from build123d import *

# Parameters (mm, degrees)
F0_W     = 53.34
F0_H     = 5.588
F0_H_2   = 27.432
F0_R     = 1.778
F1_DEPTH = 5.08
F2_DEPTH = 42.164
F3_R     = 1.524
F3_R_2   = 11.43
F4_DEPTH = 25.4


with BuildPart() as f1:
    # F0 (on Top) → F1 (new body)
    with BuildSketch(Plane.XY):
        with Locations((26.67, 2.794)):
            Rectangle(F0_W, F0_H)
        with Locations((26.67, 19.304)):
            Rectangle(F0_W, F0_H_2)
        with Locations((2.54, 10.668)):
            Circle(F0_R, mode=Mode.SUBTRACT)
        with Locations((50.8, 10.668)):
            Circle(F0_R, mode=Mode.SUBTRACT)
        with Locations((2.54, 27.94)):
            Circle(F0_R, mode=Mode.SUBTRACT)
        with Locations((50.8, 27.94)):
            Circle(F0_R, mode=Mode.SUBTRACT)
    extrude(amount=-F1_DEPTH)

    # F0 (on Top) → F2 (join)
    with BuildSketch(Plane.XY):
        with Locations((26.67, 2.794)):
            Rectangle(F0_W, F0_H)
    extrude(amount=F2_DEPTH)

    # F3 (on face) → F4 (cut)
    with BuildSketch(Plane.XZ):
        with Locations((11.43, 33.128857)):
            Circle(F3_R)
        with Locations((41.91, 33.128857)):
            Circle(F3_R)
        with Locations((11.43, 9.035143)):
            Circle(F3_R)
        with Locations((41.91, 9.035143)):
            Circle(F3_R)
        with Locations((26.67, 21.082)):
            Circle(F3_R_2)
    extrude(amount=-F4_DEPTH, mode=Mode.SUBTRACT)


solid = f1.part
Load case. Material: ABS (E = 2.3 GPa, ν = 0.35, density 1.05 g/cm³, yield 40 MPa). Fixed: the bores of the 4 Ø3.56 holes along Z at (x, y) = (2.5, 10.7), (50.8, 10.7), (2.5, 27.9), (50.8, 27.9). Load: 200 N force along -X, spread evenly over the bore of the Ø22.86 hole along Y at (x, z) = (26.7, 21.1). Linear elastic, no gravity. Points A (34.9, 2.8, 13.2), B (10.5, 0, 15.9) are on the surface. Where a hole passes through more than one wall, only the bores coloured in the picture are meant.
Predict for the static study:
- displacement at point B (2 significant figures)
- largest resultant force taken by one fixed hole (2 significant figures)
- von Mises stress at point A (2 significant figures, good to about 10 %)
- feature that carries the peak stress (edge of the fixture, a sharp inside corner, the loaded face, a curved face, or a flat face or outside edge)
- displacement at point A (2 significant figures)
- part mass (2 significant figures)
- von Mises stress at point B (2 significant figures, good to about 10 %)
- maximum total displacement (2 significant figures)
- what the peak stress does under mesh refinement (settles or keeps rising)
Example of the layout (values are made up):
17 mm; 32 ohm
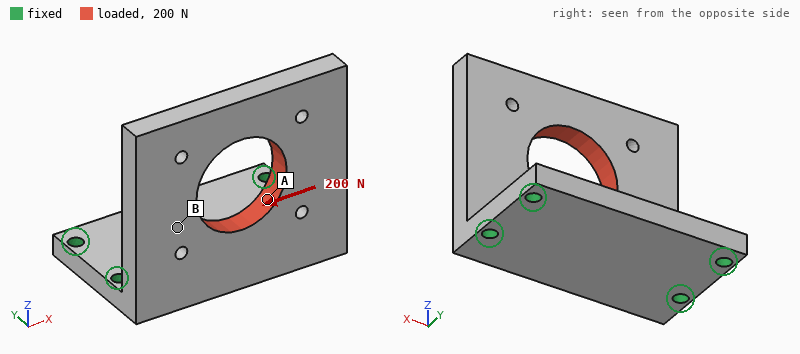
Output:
0.081 mm; 140 N; 3.8 MPa; edge of the fixture; 0.060 mm; 20 g; 1.2 MPa; 0.20 mm; keeps rising
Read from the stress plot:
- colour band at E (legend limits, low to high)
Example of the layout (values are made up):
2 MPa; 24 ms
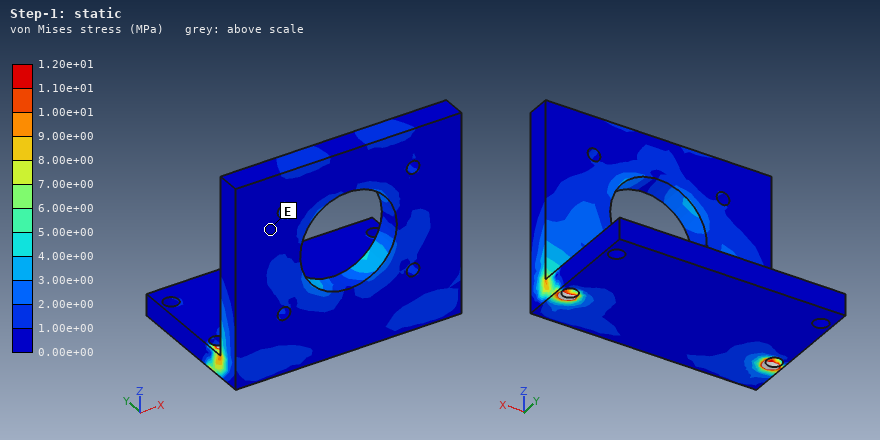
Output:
0.00e+00 to 1.00e+00 MPa
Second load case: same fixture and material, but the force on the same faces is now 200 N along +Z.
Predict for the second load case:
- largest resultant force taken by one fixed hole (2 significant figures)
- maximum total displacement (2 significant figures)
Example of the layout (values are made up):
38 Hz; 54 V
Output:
120 N; 0.33 mm
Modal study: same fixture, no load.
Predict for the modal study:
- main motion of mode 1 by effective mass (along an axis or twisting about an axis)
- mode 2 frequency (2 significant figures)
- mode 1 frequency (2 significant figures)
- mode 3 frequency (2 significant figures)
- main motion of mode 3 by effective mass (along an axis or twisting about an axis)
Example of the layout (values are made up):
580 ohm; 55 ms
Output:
along Y; 1100 Hz; 480 Hz; 2000 Hz; along X
